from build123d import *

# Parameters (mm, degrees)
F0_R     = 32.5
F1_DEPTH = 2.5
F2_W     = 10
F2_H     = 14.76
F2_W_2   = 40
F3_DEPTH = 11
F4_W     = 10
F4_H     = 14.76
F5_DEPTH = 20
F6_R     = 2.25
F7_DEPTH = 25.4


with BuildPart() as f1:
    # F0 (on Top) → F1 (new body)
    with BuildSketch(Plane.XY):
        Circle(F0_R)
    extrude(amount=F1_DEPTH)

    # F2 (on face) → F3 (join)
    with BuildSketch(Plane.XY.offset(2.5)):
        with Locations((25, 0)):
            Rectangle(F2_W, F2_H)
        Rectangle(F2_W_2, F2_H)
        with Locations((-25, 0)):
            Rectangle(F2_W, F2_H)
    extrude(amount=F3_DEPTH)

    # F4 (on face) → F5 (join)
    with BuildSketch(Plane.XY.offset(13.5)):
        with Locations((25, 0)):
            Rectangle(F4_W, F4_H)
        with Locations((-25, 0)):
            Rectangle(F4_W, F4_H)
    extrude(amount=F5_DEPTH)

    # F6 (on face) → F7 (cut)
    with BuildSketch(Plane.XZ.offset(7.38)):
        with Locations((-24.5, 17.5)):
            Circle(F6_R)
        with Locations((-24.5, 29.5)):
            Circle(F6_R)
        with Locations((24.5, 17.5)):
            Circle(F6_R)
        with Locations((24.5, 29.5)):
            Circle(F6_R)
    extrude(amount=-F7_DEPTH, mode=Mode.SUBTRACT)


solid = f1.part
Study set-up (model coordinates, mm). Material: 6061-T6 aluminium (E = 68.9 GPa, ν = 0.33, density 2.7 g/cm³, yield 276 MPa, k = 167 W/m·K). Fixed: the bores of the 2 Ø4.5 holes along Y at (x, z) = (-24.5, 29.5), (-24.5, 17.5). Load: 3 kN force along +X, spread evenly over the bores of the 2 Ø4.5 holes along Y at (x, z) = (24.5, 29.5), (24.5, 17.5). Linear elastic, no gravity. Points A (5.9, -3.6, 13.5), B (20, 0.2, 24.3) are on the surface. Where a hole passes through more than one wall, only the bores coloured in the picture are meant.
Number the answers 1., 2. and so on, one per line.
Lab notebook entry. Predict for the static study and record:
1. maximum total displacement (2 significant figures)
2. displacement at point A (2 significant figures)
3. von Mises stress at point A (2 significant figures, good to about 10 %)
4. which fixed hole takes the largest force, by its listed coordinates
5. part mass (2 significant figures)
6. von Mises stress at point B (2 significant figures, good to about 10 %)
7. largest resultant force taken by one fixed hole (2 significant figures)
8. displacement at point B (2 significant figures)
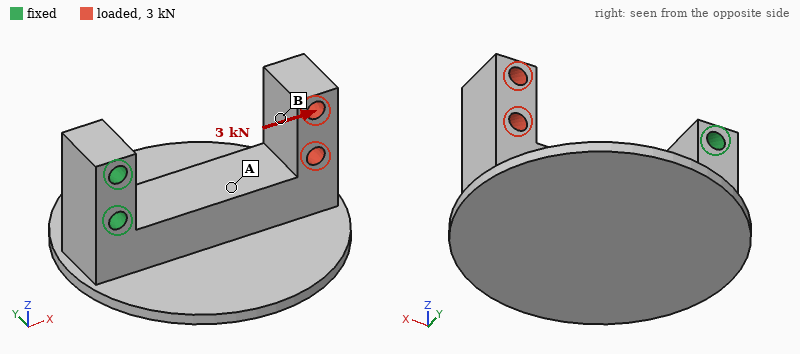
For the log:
1. 0.61 mm
2. 0.18 mm
3. 110 MPa
4. (-24.5, 17.5)
5. 62 g
6. 36 MPa
7. 2.5 kN
8. 0.39 mm
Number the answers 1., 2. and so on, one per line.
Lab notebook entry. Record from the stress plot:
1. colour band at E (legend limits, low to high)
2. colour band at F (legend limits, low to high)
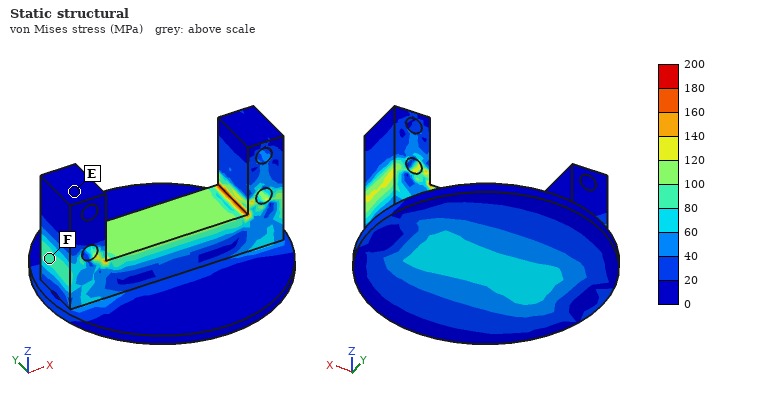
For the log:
1. 0 to 20 MPa
2. 80 to 100 MPa
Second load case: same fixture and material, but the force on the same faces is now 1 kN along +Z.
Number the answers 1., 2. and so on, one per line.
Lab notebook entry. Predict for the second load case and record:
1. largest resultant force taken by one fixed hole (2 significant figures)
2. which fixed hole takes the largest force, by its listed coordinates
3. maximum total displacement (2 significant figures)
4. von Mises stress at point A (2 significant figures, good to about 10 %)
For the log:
1. 1.9 kN
2. (-24.5, 17.5)
3. 0.51 mm
4. 34 MPa
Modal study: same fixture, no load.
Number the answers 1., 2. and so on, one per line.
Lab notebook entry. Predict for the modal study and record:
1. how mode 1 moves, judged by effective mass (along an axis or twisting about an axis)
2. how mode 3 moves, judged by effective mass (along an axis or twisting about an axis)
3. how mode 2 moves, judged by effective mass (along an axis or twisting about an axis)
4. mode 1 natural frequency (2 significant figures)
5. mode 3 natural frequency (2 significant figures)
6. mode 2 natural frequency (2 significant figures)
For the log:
1. along Z
2. twisting about X
3. along Y
4. 1600 Hz
5. 3100 Hz
6. 2000 Hz
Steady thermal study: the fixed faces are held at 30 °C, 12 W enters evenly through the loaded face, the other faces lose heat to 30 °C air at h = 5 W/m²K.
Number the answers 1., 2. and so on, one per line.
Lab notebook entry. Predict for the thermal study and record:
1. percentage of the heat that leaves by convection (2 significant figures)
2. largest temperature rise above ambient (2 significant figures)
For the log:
1. 4.2 %
2. 24 K
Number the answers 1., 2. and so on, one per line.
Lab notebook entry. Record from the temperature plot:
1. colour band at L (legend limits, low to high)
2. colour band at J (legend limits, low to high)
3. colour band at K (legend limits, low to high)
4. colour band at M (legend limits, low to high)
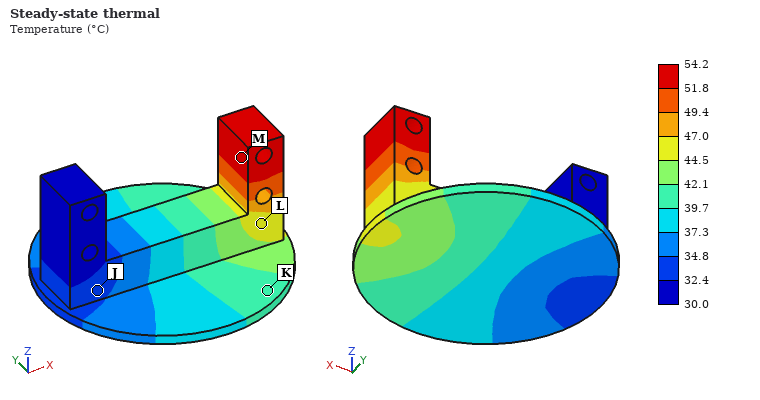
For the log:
1. 44.5 to 47.0 °C
2. 32.4 to 34.8 °C
3. 39.7 to 42.1 °C
4. 51.8 to 54.2 °C
